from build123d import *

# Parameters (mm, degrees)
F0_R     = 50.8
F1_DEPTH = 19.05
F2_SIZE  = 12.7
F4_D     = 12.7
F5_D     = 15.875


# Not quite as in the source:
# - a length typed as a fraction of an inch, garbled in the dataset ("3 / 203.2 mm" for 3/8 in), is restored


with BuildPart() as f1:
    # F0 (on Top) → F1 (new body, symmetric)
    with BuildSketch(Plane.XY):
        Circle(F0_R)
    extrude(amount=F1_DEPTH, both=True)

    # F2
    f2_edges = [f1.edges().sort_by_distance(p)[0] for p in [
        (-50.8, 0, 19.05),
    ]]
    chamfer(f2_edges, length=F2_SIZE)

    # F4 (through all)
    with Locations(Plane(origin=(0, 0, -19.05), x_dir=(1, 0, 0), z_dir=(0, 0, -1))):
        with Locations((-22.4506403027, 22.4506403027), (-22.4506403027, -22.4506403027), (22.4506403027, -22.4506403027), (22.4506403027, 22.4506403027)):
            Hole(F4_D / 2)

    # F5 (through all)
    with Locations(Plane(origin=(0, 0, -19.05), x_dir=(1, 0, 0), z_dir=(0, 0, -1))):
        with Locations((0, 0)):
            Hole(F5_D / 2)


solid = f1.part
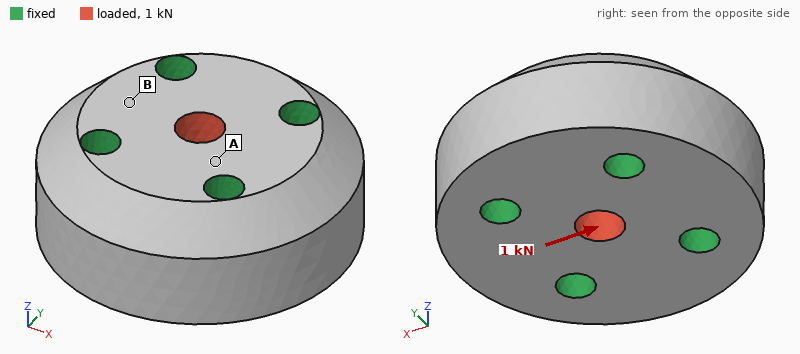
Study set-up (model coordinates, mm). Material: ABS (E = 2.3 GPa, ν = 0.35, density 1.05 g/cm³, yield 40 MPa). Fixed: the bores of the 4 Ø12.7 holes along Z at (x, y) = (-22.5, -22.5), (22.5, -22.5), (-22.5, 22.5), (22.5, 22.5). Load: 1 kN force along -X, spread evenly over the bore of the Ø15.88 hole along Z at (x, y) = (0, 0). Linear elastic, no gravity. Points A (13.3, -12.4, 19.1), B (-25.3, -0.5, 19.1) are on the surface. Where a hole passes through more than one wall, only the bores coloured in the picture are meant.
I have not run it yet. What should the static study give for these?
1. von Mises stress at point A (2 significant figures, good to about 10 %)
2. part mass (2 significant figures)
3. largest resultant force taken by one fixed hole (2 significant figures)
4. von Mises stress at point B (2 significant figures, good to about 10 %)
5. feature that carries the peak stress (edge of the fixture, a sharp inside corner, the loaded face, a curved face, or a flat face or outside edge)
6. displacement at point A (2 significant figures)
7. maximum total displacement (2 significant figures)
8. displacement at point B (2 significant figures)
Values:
0.41 MPa
270 g
270 N
0.16 MPa
the loaded face
1.8 µm
5.0 µm
2.5 µm
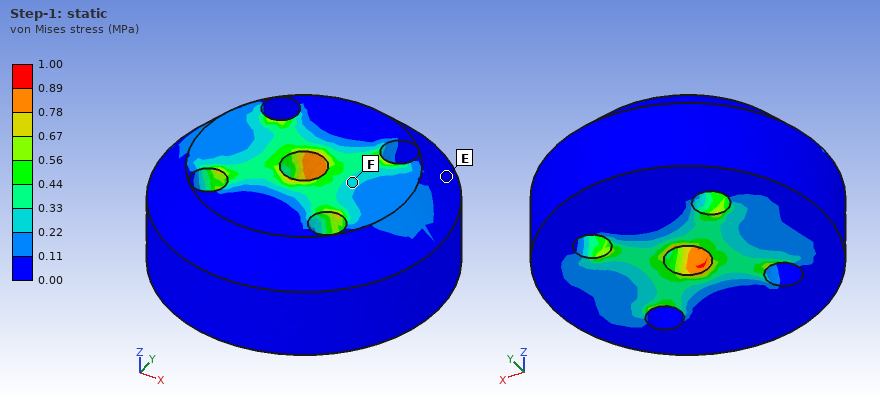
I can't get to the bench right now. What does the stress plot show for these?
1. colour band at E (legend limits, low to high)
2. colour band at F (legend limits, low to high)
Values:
0.00 to 0.11 MPa
0.22 to 0.33 MPa
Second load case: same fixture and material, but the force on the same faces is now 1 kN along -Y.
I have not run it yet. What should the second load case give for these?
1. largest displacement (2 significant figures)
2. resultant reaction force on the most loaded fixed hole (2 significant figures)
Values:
5.1 µm
270 N
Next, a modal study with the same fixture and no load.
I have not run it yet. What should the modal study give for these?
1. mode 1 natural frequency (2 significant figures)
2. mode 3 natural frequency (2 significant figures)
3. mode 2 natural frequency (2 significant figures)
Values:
7300 Hz
7400 Hz
7400 Hz
